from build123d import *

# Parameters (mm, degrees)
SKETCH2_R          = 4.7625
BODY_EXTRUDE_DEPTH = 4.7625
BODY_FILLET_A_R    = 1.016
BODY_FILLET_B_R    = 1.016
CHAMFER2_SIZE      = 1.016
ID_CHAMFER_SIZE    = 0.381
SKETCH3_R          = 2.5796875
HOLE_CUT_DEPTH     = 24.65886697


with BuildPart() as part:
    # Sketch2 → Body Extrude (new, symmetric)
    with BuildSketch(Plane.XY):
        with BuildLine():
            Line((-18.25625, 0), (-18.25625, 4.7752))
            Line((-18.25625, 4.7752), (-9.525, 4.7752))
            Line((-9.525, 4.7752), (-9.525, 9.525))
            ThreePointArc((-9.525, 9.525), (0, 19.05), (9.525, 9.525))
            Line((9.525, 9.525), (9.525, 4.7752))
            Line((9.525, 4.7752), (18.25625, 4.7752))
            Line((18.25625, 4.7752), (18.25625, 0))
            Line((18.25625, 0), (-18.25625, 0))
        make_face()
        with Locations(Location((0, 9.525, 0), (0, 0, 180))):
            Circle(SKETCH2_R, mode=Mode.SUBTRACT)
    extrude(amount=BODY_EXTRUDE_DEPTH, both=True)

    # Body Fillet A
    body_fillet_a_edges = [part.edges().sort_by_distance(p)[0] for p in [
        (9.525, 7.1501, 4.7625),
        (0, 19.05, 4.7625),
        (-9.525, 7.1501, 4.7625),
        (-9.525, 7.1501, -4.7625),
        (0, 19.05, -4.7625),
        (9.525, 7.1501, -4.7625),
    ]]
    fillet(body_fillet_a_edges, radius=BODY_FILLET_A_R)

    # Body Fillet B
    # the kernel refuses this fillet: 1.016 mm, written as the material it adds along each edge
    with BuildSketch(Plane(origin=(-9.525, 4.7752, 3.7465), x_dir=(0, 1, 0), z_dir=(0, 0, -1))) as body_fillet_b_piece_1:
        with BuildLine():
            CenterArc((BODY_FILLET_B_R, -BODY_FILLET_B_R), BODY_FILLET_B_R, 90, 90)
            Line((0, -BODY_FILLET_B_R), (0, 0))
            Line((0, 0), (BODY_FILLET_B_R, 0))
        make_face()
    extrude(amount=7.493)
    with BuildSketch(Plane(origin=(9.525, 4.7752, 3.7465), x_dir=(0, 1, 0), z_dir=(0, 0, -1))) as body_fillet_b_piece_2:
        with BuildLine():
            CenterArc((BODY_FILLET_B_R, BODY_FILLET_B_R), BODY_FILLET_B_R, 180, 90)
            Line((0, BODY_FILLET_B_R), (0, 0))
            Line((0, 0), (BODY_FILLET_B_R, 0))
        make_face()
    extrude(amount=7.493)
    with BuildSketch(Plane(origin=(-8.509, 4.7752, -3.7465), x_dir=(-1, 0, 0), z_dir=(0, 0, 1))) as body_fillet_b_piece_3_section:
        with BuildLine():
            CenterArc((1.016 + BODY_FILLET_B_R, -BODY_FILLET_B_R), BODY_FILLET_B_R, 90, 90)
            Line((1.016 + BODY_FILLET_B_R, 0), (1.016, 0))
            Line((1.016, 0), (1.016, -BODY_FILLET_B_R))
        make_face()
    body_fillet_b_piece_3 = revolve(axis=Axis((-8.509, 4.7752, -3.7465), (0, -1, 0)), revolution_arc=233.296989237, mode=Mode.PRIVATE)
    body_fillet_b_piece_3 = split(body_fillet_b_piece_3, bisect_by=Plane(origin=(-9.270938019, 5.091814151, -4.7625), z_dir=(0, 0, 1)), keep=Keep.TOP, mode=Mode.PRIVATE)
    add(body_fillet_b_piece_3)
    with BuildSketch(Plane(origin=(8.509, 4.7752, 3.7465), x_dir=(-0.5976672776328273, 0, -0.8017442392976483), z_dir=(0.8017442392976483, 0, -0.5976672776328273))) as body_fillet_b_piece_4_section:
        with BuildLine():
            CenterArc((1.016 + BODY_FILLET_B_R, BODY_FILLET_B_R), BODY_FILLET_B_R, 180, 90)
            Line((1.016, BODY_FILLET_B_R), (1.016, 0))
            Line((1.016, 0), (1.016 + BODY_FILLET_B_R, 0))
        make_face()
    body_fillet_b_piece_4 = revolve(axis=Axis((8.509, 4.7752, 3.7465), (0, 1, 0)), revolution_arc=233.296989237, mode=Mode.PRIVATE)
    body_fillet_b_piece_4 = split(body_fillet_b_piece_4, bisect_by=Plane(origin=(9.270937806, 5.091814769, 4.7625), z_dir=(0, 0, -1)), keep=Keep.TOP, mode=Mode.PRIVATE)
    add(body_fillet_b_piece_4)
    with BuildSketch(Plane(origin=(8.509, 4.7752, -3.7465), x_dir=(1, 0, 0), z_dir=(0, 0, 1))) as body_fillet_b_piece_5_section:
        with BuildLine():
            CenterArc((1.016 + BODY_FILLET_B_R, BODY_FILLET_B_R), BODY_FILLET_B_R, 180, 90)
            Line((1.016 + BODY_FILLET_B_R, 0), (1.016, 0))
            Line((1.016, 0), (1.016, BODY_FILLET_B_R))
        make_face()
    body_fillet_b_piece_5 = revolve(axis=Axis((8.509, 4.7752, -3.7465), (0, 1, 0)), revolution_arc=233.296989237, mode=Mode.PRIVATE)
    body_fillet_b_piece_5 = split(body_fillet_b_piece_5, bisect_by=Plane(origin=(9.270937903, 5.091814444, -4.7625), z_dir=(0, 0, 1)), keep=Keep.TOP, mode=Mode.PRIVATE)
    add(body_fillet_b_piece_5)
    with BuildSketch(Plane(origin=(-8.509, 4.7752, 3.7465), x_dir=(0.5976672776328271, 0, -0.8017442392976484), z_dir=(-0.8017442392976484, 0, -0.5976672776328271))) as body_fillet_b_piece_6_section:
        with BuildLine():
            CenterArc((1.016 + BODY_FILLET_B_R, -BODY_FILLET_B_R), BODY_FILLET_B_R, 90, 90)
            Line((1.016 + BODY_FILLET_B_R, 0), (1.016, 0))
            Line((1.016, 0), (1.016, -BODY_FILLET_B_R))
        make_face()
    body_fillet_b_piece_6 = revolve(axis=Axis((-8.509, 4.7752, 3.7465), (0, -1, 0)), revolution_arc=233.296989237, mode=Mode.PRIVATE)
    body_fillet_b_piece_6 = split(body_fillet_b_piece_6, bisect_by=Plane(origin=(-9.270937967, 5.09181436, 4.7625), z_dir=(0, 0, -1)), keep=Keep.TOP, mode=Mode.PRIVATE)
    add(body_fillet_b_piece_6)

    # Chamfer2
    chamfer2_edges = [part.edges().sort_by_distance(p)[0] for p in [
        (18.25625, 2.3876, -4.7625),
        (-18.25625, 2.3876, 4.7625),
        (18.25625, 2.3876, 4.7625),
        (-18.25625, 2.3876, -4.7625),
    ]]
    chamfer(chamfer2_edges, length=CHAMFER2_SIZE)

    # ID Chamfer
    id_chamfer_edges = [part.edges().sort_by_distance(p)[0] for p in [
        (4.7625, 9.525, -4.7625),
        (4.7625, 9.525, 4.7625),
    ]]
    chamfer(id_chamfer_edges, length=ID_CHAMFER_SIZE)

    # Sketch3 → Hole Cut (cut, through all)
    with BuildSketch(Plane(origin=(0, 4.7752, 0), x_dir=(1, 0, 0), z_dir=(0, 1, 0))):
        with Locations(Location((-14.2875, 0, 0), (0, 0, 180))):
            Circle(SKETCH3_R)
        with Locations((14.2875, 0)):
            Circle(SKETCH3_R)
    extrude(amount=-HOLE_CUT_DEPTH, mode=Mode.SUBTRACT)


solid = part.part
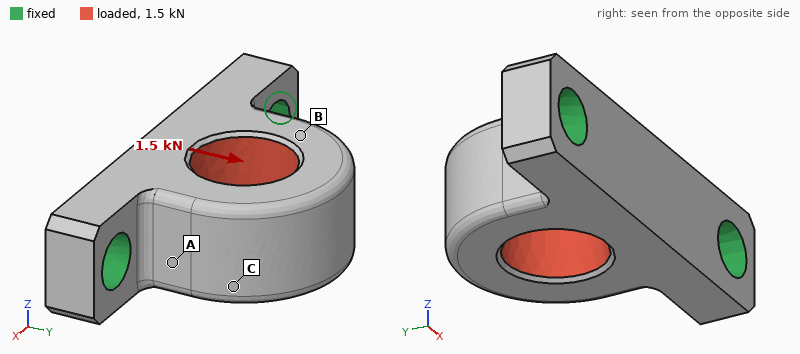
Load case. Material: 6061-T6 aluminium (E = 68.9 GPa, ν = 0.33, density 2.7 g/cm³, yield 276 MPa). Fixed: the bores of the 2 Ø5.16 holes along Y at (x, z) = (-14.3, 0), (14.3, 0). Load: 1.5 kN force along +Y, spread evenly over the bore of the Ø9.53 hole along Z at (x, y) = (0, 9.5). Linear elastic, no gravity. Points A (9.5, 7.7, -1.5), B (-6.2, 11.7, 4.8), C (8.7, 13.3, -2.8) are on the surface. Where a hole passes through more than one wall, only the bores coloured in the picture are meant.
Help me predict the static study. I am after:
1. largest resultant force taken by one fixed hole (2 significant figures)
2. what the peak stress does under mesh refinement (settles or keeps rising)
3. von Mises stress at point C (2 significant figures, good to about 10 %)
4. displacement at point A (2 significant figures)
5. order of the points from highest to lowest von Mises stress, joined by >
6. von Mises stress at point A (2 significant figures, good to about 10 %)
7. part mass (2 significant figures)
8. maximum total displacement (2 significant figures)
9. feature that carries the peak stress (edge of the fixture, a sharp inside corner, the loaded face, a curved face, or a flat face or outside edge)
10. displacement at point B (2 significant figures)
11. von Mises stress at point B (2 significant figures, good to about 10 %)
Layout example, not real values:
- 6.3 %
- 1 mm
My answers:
- 790 N
- keeps rising
- 7.3 MPa
- 5.7 µm
- A > B > C
- 28 MPa
- 8.0 g
- 8.9 µm
- edge of the fixture
- 6.6 µm
- 14 MPa
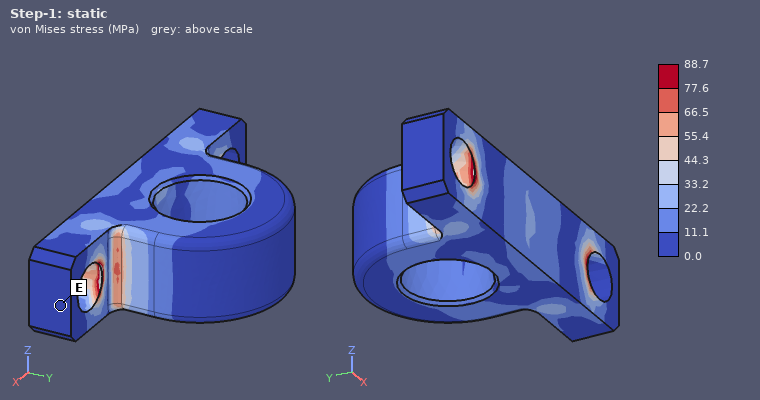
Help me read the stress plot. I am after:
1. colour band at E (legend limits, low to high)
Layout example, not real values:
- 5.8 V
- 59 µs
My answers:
- 0.0 to 11.1 MPa
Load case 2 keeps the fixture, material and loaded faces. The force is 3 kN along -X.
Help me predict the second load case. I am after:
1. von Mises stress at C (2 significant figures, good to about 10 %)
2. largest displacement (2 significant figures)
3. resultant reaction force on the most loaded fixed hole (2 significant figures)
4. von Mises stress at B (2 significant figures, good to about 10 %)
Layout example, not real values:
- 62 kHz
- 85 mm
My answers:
- 24 MPa
- 24 µm
- 1.8 kN
- 35 MPa
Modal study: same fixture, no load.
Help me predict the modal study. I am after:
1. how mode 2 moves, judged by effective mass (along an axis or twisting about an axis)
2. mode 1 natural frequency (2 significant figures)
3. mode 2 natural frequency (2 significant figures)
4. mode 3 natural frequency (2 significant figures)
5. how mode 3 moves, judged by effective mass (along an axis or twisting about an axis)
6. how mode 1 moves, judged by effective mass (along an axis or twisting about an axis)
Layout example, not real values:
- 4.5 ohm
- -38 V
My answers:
- along X
- 12 kHz
- 27 kHz
- 30 kHz
- along Y
- along Z
